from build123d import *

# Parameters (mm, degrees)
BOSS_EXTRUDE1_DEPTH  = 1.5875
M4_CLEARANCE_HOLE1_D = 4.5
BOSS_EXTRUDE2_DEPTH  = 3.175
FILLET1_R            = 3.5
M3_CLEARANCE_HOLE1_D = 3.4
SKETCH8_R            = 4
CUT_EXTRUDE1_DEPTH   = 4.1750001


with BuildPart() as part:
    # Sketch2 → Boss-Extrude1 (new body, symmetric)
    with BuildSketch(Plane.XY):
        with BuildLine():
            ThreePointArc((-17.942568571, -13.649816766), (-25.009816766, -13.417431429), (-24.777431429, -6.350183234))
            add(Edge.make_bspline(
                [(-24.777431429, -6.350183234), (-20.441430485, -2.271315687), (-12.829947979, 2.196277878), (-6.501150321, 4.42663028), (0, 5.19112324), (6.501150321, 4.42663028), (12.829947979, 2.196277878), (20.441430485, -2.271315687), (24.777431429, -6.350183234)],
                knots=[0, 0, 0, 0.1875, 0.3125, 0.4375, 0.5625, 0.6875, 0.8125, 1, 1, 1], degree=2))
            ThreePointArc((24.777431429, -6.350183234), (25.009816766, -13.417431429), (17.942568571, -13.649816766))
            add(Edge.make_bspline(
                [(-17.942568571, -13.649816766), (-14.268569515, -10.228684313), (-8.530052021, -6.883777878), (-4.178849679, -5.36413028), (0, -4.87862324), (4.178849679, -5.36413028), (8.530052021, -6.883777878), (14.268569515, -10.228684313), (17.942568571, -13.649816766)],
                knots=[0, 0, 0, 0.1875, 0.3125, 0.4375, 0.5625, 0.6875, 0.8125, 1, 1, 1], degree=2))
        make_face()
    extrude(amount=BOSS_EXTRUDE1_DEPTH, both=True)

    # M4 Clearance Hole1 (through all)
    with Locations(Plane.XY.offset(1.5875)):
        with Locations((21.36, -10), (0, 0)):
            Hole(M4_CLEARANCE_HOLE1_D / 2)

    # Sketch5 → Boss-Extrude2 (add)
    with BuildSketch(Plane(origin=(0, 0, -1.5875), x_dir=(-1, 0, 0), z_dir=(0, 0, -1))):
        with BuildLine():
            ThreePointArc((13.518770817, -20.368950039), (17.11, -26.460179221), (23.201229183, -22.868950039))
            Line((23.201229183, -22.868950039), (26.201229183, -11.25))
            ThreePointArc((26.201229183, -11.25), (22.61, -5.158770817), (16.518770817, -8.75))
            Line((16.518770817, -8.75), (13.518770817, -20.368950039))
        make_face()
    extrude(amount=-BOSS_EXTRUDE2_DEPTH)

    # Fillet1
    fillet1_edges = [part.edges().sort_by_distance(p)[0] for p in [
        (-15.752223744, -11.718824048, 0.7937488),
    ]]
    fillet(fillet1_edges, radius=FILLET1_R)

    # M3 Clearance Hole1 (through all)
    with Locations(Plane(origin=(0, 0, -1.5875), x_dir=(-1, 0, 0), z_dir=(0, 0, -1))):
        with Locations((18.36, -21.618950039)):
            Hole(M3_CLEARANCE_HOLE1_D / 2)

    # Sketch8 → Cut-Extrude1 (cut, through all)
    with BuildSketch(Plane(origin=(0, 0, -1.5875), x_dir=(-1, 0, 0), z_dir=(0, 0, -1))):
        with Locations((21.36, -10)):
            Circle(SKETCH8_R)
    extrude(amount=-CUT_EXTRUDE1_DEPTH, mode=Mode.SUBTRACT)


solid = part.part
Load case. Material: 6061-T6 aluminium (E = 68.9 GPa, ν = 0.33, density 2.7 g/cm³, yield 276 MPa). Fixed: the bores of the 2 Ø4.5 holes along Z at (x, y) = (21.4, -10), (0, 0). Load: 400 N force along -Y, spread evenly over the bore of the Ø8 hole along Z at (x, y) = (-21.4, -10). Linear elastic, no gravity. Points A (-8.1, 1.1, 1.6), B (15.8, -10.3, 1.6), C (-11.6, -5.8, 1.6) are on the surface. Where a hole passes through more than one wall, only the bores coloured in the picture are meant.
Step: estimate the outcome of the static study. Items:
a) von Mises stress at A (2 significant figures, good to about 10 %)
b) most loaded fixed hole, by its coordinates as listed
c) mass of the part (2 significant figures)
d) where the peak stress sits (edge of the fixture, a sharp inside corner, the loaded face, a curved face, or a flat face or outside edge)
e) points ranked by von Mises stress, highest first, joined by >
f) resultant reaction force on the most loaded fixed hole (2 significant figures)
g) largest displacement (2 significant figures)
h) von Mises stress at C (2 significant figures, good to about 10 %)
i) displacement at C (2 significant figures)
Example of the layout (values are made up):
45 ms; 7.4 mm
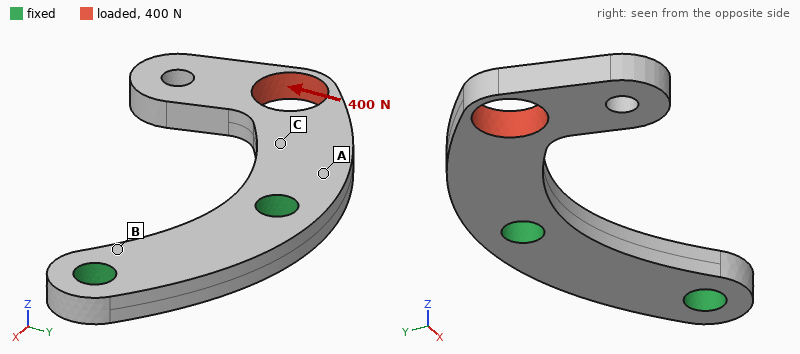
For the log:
63 MPa; (0, 0); 5.1 g; edge of the fixture; A > C > B; 500 N; 0.23 mm; 35 MPa; 0.045 mm
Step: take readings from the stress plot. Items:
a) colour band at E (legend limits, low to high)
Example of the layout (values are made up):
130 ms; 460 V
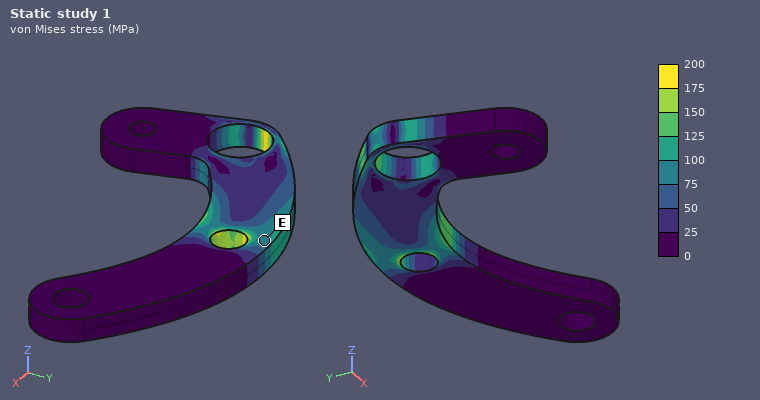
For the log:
75 to 100 MPa
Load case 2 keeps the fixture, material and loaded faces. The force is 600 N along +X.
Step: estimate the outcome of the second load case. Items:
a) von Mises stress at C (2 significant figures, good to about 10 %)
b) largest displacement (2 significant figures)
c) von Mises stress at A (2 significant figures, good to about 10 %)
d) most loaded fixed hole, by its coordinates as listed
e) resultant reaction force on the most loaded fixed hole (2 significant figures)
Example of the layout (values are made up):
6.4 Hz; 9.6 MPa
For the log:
50 MPa; 0.21 mm; 36 MPa; (0, 0); 590 N
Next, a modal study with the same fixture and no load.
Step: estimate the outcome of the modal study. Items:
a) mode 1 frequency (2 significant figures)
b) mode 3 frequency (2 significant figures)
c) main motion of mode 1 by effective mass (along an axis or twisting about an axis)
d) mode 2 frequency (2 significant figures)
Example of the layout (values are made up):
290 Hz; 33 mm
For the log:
2300 Hz; 6700 Hz; along Z; 5300 Hz
